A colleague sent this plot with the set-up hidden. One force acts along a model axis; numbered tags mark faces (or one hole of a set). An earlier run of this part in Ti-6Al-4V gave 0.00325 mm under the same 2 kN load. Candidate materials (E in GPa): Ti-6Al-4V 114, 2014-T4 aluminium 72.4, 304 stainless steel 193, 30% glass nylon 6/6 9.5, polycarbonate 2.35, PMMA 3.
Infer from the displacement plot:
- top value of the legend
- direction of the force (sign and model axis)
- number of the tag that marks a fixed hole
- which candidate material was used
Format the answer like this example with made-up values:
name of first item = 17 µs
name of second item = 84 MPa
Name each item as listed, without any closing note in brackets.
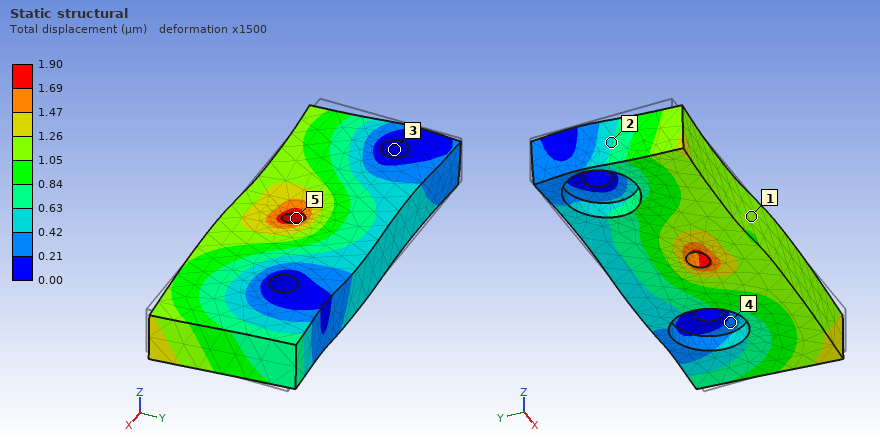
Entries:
top value of the legend = 1.90 µm
direction of the force = +X
number of the tag that marks a fixed hole = 3
which candidate material was used = 304 stainless steel
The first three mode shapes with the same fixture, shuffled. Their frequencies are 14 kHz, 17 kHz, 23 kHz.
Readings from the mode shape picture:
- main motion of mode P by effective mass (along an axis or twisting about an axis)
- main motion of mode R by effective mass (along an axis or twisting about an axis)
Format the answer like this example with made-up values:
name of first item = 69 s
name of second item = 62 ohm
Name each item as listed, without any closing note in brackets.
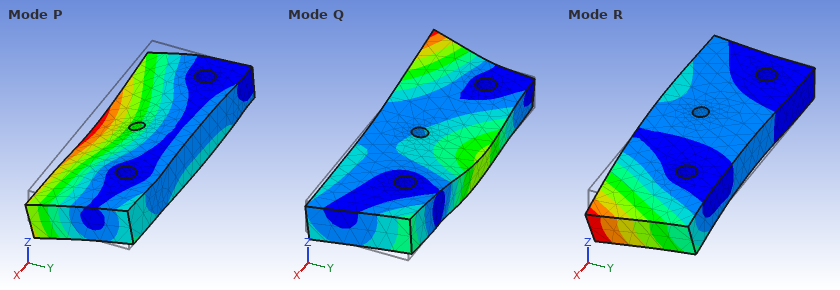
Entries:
main motion of mode P by effective mass = along Z
main motion of mode R by effective mass = twisting about Y
